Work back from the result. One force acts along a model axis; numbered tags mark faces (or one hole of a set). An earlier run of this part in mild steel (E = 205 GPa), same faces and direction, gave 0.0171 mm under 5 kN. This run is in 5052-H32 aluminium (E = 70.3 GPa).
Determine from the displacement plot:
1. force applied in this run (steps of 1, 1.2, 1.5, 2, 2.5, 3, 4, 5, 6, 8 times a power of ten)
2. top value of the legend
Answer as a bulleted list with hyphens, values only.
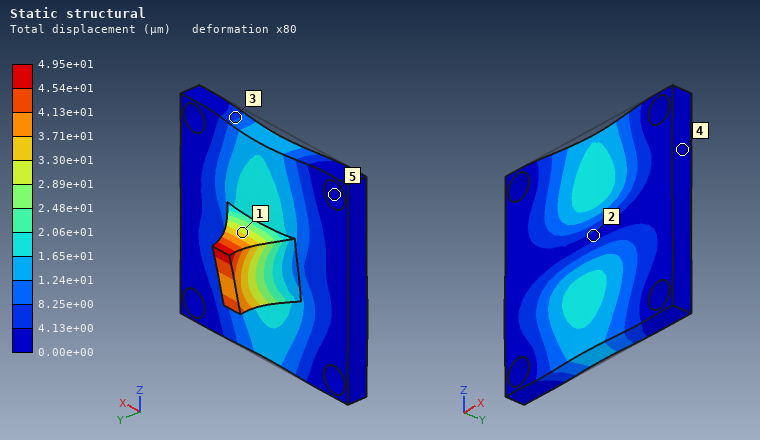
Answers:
- 5 kN
- 4.95e+01 µm
